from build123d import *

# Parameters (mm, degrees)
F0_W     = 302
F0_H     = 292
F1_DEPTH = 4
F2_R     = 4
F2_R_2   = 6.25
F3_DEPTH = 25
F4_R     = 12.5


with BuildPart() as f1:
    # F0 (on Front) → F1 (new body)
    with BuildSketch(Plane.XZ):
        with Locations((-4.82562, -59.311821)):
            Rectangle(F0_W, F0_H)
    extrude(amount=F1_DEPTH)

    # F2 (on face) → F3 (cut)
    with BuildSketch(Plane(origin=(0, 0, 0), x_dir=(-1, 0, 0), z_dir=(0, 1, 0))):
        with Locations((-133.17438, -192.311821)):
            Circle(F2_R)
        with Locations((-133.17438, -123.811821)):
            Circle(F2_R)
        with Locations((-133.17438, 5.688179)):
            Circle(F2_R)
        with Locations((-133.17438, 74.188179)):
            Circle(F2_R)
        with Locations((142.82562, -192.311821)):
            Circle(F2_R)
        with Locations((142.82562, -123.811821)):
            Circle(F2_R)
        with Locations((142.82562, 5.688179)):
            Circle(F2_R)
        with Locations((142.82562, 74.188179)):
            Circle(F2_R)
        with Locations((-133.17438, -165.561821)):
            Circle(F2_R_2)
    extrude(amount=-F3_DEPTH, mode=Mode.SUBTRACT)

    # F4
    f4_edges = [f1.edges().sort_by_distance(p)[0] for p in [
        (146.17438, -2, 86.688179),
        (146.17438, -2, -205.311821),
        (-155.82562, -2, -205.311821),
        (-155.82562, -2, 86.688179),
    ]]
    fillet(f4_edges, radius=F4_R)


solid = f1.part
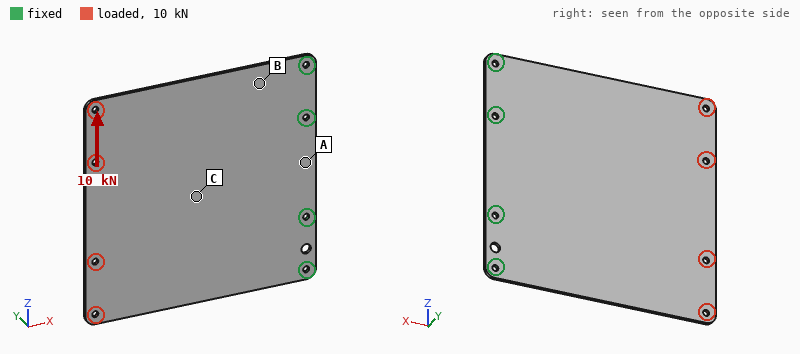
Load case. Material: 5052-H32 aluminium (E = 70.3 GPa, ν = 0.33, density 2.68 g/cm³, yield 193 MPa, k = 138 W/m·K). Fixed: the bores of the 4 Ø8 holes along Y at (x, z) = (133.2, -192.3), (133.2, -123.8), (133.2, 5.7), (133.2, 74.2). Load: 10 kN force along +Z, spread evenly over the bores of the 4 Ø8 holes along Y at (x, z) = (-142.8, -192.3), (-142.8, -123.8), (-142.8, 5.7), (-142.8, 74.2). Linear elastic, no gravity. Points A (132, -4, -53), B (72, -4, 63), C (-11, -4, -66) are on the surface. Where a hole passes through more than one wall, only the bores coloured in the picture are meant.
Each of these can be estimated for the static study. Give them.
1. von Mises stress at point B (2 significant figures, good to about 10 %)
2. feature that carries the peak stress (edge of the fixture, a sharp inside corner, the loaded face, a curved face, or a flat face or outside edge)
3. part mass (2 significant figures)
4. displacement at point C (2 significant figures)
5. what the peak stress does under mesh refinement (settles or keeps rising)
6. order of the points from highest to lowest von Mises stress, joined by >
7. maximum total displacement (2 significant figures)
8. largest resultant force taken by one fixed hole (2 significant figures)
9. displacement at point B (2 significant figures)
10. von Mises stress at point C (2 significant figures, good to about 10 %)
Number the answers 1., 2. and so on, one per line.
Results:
1. 34 MPa
2. edge of the fixture
3. 940 g
4. 0.10 mm
5. keeps rising
6. B > C > A
7. 0.30 mm
8. 8.6 kN
9. 0.057 mm
10. 23 MPa
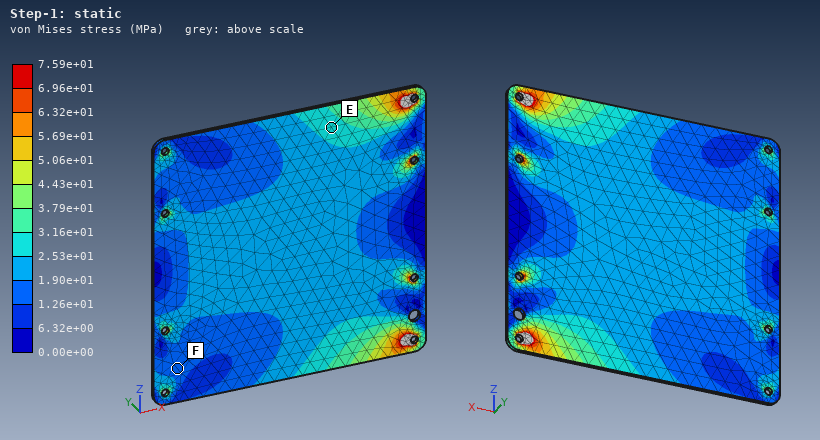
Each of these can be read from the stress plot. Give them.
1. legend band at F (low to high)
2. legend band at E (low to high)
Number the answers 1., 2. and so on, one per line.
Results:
1. 1.26e+01 to 1.90e+01 MPa
2. 2.53e+01 to 3.16e+01 MPa
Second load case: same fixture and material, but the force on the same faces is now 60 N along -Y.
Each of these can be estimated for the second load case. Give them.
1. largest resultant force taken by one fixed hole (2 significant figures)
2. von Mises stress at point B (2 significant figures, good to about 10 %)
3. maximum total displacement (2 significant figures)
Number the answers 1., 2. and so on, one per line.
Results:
1. 42 N
2. 17 MPa
3. 4.3 mm
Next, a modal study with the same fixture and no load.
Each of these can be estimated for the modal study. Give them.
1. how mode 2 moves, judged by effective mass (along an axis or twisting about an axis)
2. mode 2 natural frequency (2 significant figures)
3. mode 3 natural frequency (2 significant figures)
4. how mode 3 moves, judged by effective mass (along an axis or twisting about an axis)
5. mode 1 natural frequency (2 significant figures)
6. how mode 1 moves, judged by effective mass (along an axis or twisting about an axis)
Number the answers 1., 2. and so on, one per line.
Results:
1. twisting about X
2. 99 Hz
3. 240 Hz
4. along Y
5. 39 Hz
6. along Y
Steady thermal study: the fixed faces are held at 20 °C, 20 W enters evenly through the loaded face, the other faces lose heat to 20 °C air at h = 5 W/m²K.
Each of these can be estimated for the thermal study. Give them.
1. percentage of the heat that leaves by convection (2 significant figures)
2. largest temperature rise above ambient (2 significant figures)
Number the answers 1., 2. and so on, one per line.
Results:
1. 51 %
2. 29 K
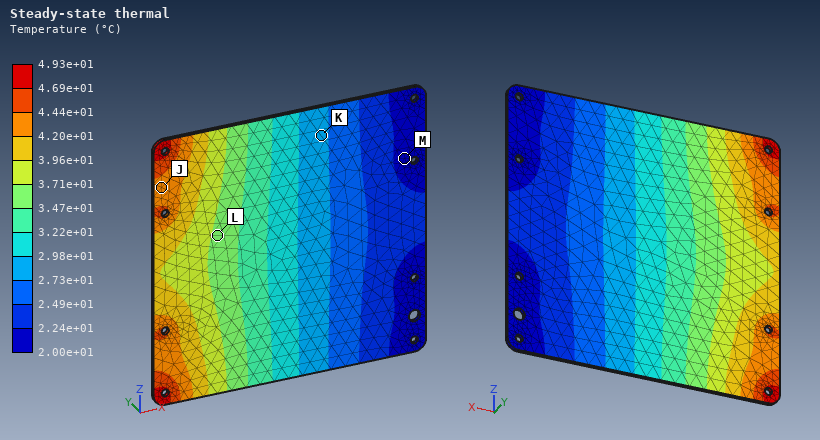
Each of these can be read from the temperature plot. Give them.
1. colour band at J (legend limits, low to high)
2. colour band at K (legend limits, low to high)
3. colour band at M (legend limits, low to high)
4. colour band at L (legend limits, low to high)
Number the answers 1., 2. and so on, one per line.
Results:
1. 4.20e+01 to 4.44e+01 °C
2. 2.73e+01 to 2.98e+01 °C
3. 2.00e+01 to 2.24e+01 °C
4. 3.47e+01 to 3.71e+01 °C
